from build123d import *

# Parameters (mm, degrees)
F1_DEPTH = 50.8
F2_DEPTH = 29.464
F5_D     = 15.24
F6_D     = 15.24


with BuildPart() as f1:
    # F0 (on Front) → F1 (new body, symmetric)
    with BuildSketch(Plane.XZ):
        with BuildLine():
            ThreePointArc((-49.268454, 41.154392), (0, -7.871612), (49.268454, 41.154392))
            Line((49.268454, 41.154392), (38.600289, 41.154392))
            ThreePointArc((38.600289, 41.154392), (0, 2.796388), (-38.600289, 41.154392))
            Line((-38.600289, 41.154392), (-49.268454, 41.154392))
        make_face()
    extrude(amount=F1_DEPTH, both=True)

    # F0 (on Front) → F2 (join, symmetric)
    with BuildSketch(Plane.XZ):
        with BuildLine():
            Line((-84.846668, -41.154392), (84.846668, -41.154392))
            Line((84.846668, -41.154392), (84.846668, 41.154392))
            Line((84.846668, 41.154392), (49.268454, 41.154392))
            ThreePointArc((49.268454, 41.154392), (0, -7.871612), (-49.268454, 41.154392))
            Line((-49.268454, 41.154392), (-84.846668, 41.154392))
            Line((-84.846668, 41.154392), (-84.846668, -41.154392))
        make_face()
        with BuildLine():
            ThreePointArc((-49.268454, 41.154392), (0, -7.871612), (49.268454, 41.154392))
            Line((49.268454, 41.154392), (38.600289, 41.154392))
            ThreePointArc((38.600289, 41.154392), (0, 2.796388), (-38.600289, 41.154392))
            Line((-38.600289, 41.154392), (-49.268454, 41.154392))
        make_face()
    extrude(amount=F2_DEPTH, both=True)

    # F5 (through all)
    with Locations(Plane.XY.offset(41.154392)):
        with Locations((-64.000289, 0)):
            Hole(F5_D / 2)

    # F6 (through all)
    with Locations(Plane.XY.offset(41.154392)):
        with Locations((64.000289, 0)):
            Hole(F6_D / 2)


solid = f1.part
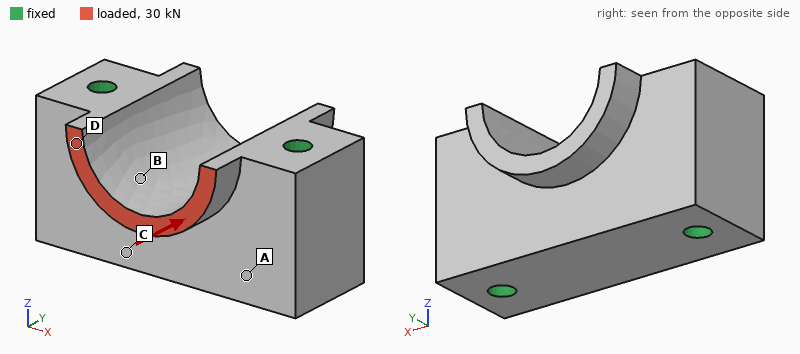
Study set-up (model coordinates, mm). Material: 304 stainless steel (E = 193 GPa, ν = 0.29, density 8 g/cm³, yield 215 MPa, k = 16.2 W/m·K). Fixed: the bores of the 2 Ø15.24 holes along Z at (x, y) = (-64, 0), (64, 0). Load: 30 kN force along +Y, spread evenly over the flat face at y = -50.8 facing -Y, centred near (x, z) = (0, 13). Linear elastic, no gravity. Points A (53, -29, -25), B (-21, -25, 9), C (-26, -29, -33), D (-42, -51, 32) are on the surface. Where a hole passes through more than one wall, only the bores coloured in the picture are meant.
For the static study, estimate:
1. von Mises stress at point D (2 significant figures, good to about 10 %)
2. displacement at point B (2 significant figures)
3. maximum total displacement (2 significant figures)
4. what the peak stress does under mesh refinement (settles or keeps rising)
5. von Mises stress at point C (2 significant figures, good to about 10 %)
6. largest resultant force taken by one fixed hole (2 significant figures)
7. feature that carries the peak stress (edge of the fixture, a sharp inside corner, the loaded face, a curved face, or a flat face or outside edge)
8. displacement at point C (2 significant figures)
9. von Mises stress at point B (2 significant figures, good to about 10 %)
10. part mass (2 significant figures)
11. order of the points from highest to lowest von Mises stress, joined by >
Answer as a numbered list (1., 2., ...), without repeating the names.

1. 20 MPa
2. 4.4 µm
3. 8.8 µm
4. keeps rising
5. 4.5 MPa
6. 15 kN
7. edge of the fixture
8. 2.1 µm
9. 10 MPa
10. 5.8 kg
11. D > B > C > A
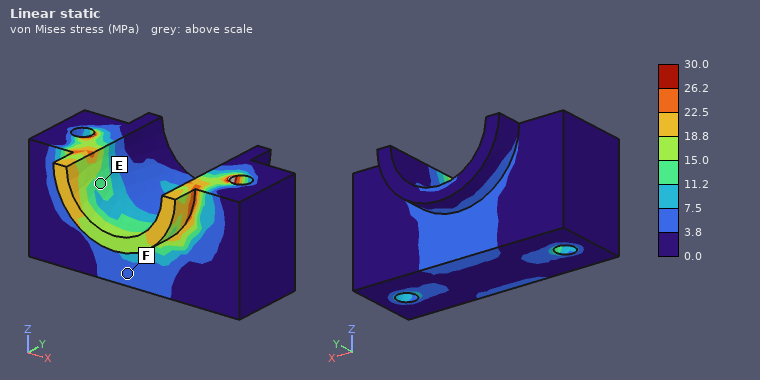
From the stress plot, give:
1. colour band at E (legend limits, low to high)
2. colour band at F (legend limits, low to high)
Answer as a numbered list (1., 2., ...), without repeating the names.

1. 11.2 to 15.0 MPa
2. 3.8 to 7.5 MPa
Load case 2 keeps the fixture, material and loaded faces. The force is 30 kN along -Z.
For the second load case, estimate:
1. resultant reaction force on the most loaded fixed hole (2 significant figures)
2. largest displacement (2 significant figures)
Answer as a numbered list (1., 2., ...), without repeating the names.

1. 16 kN
2. 43 µm
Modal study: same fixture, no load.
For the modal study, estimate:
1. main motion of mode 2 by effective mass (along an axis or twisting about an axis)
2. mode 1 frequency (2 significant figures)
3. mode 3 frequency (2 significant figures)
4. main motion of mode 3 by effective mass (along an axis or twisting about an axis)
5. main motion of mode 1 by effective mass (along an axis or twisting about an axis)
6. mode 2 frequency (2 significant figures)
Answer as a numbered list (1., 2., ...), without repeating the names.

1. along Z
2. 8000 Hz
3. 11 kHz
4. twisting about X
5. along Y
6. 10 kHz
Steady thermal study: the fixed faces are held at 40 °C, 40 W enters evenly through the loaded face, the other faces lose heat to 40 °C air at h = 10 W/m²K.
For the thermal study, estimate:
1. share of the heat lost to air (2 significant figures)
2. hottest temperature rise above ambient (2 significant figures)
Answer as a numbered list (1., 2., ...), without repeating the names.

1. 12 %
2. 58 K
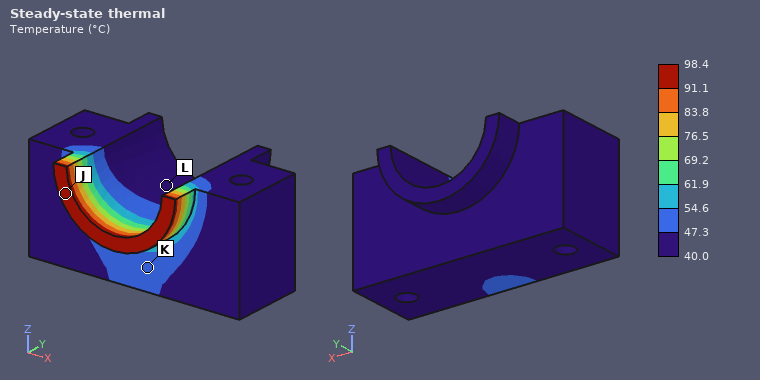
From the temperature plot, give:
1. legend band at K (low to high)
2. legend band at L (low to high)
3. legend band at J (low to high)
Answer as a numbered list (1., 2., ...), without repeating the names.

1. 47.3 to 54.6 °C
2. 40.0 to 47.3 °C
3. 91.1 to 98.4 °C
